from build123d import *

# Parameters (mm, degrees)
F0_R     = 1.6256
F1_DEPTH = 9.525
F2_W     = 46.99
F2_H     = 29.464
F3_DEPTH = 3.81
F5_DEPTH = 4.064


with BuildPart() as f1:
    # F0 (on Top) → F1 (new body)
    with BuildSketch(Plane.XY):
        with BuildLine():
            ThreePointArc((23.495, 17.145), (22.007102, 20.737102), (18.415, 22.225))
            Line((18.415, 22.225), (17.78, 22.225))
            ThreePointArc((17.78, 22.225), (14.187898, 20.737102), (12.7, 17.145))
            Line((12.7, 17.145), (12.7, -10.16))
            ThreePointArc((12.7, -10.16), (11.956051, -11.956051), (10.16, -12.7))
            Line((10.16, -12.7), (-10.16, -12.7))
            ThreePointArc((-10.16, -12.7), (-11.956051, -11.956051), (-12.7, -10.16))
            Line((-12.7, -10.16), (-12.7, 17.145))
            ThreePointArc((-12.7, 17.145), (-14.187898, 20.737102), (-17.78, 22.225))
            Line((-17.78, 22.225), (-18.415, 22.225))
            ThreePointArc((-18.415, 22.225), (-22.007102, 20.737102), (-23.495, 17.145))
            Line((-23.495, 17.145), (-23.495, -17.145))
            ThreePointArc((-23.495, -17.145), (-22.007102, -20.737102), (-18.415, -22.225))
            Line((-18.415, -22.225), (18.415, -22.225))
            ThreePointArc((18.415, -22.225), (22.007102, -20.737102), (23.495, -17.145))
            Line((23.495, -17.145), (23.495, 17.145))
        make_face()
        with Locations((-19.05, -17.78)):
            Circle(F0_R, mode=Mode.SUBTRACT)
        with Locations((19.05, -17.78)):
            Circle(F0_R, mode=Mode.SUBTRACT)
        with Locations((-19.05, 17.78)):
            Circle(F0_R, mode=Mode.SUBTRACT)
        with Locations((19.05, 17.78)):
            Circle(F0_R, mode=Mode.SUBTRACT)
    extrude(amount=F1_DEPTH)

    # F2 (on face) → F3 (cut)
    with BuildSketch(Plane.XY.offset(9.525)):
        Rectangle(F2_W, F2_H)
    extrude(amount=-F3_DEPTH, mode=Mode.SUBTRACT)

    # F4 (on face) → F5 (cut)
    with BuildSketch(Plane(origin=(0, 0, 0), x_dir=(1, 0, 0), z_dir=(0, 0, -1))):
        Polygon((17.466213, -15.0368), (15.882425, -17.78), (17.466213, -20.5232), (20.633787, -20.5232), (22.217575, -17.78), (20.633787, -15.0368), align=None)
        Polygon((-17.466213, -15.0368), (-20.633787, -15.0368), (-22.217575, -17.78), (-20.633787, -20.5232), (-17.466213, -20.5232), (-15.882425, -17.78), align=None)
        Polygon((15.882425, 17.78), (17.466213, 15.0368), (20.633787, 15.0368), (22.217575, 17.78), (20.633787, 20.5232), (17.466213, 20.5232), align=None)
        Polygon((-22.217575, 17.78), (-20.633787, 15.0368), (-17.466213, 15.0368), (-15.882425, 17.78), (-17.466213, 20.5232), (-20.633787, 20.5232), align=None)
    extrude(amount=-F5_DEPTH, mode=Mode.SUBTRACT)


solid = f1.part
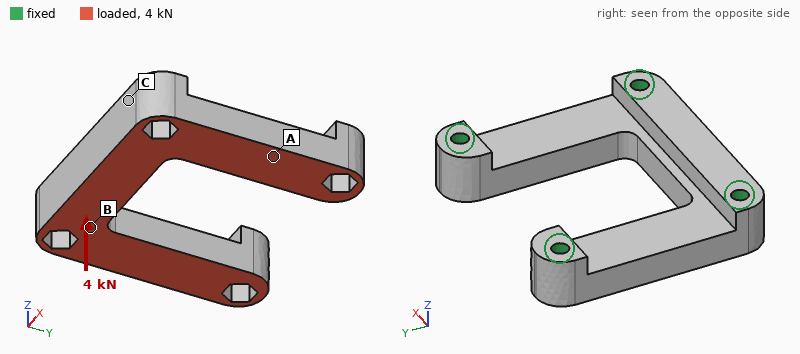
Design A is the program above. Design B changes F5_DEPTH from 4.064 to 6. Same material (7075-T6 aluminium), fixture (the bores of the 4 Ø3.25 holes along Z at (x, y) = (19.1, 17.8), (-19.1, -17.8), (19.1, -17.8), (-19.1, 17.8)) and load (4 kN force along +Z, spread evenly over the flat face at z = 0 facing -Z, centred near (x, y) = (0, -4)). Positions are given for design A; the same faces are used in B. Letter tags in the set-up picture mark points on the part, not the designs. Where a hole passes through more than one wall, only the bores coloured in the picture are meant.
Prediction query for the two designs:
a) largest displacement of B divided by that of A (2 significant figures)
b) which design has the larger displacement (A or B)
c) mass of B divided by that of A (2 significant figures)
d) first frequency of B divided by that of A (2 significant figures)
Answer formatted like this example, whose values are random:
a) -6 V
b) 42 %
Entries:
a) 1.2
b) B
c) 0.98
d) 0.90
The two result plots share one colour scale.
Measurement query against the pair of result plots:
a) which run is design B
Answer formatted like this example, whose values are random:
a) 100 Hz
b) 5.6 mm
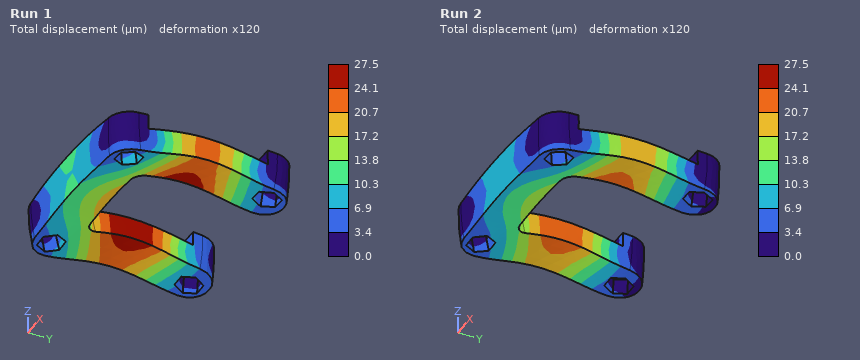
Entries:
a) Run 1
